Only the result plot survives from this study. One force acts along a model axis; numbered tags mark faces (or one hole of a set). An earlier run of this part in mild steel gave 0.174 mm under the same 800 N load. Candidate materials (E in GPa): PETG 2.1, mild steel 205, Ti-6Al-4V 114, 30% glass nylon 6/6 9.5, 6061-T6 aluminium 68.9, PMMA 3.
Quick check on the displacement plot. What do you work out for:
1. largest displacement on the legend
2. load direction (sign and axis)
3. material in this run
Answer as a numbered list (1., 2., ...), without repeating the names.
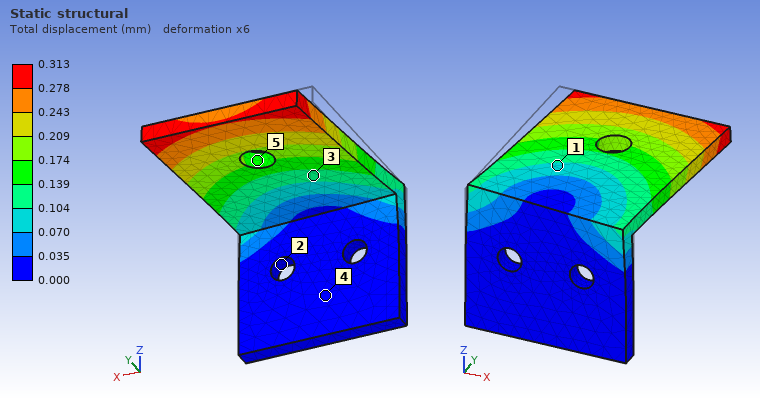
1. 0.313 mm
2. +X
3. Ti-6Al-4V
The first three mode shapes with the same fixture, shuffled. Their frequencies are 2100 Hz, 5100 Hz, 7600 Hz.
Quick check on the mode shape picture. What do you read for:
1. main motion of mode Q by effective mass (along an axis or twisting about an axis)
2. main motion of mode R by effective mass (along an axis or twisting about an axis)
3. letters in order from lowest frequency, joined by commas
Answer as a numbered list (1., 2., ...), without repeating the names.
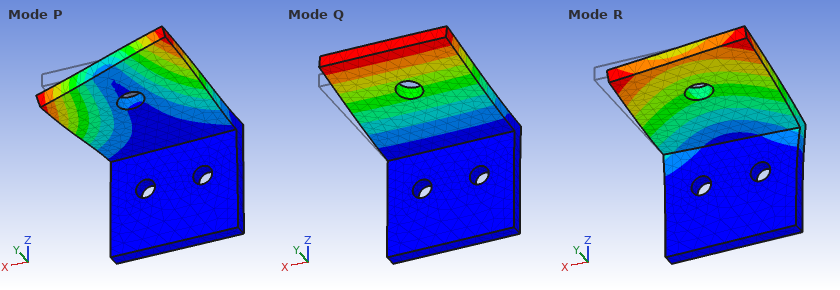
1. along Z
2. along X
3. Q, R, P
